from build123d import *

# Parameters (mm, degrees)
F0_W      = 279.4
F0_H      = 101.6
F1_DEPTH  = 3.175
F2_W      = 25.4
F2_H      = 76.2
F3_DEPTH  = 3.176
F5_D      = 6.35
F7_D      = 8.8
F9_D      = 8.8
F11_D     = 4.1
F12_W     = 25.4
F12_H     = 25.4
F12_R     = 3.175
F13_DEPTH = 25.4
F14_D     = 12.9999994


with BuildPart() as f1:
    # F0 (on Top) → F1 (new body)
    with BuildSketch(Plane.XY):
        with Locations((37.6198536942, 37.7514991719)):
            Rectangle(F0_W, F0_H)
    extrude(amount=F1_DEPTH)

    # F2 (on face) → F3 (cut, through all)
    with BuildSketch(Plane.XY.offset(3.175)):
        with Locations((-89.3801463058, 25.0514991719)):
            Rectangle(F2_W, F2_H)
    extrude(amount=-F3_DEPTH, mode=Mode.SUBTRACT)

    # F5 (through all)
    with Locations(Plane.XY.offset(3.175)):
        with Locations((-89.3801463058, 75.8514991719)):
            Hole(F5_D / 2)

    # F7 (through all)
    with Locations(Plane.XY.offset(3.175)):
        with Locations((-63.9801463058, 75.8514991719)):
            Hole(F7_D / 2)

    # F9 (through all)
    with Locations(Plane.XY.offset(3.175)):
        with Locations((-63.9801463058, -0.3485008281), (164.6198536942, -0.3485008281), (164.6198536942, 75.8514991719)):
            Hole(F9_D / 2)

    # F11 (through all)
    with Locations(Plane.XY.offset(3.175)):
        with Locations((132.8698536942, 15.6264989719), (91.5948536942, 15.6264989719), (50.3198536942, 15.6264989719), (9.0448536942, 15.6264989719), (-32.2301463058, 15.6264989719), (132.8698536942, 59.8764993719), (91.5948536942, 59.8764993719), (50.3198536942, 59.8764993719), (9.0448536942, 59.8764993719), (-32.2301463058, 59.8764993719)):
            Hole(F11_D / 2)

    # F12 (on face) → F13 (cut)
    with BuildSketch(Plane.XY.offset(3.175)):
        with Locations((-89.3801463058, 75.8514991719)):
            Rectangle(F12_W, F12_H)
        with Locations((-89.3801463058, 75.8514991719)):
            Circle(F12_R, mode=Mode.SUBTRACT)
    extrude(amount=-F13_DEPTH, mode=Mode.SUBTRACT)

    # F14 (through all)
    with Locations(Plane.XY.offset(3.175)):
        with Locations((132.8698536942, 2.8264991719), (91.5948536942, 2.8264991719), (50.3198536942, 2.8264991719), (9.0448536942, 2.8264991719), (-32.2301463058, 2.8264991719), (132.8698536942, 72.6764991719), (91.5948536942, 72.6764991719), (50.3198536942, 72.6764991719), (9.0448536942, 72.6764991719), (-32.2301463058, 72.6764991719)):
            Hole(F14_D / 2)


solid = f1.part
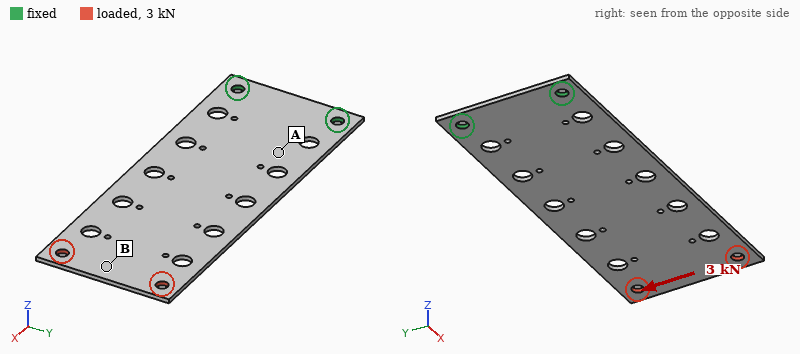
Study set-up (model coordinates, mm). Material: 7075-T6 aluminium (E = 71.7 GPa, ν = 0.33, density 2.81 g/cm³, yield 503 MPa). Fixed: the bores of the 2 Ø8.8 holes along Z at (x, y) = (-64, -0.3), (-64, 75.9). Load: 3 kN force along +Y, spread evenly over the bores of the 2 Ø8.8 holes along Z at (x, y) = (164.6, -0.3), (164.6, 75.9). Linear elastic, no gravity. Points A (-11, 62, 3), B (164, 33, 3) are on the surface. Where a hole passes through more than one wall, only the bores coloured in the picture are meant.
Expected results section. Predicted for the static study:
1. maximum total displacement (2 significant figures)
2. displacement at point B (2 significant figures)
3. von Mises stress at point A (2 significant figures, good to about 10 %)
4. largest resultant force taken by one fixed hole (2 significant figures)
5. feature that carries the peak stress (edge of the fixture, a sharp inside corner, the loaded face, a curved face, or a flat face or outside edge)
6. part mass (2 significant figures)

1.0 mm
0.90 mm
49 MPa
8.8 kN
a curved face
220 g
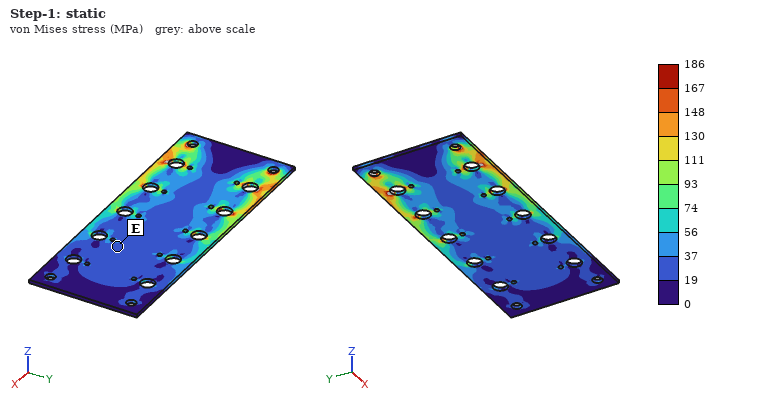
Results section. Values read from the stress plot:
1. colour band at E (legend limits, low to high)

19 to 37 MPa
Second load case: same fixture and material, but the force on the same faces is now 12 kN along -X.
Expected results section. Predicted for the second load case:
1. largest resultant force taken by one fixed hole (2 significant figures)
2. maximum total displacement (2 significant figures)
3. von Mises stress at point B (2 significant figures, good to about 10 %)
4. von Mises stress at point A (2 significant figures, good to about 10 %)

6.1 kN
0.19 mm
19 MPa
34 MPa
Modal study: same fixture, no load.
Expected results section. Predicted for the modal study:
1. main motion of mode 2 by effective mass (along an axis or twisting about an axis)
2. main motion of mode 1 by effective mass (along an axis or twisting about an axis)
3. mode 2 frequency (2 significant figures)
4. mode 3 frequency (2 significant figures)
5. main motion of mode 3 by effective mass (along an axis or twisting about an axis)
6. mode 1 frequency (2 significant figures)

twisting about X
along Z
230 Hz
270 Hz
along Z
43 Hz
